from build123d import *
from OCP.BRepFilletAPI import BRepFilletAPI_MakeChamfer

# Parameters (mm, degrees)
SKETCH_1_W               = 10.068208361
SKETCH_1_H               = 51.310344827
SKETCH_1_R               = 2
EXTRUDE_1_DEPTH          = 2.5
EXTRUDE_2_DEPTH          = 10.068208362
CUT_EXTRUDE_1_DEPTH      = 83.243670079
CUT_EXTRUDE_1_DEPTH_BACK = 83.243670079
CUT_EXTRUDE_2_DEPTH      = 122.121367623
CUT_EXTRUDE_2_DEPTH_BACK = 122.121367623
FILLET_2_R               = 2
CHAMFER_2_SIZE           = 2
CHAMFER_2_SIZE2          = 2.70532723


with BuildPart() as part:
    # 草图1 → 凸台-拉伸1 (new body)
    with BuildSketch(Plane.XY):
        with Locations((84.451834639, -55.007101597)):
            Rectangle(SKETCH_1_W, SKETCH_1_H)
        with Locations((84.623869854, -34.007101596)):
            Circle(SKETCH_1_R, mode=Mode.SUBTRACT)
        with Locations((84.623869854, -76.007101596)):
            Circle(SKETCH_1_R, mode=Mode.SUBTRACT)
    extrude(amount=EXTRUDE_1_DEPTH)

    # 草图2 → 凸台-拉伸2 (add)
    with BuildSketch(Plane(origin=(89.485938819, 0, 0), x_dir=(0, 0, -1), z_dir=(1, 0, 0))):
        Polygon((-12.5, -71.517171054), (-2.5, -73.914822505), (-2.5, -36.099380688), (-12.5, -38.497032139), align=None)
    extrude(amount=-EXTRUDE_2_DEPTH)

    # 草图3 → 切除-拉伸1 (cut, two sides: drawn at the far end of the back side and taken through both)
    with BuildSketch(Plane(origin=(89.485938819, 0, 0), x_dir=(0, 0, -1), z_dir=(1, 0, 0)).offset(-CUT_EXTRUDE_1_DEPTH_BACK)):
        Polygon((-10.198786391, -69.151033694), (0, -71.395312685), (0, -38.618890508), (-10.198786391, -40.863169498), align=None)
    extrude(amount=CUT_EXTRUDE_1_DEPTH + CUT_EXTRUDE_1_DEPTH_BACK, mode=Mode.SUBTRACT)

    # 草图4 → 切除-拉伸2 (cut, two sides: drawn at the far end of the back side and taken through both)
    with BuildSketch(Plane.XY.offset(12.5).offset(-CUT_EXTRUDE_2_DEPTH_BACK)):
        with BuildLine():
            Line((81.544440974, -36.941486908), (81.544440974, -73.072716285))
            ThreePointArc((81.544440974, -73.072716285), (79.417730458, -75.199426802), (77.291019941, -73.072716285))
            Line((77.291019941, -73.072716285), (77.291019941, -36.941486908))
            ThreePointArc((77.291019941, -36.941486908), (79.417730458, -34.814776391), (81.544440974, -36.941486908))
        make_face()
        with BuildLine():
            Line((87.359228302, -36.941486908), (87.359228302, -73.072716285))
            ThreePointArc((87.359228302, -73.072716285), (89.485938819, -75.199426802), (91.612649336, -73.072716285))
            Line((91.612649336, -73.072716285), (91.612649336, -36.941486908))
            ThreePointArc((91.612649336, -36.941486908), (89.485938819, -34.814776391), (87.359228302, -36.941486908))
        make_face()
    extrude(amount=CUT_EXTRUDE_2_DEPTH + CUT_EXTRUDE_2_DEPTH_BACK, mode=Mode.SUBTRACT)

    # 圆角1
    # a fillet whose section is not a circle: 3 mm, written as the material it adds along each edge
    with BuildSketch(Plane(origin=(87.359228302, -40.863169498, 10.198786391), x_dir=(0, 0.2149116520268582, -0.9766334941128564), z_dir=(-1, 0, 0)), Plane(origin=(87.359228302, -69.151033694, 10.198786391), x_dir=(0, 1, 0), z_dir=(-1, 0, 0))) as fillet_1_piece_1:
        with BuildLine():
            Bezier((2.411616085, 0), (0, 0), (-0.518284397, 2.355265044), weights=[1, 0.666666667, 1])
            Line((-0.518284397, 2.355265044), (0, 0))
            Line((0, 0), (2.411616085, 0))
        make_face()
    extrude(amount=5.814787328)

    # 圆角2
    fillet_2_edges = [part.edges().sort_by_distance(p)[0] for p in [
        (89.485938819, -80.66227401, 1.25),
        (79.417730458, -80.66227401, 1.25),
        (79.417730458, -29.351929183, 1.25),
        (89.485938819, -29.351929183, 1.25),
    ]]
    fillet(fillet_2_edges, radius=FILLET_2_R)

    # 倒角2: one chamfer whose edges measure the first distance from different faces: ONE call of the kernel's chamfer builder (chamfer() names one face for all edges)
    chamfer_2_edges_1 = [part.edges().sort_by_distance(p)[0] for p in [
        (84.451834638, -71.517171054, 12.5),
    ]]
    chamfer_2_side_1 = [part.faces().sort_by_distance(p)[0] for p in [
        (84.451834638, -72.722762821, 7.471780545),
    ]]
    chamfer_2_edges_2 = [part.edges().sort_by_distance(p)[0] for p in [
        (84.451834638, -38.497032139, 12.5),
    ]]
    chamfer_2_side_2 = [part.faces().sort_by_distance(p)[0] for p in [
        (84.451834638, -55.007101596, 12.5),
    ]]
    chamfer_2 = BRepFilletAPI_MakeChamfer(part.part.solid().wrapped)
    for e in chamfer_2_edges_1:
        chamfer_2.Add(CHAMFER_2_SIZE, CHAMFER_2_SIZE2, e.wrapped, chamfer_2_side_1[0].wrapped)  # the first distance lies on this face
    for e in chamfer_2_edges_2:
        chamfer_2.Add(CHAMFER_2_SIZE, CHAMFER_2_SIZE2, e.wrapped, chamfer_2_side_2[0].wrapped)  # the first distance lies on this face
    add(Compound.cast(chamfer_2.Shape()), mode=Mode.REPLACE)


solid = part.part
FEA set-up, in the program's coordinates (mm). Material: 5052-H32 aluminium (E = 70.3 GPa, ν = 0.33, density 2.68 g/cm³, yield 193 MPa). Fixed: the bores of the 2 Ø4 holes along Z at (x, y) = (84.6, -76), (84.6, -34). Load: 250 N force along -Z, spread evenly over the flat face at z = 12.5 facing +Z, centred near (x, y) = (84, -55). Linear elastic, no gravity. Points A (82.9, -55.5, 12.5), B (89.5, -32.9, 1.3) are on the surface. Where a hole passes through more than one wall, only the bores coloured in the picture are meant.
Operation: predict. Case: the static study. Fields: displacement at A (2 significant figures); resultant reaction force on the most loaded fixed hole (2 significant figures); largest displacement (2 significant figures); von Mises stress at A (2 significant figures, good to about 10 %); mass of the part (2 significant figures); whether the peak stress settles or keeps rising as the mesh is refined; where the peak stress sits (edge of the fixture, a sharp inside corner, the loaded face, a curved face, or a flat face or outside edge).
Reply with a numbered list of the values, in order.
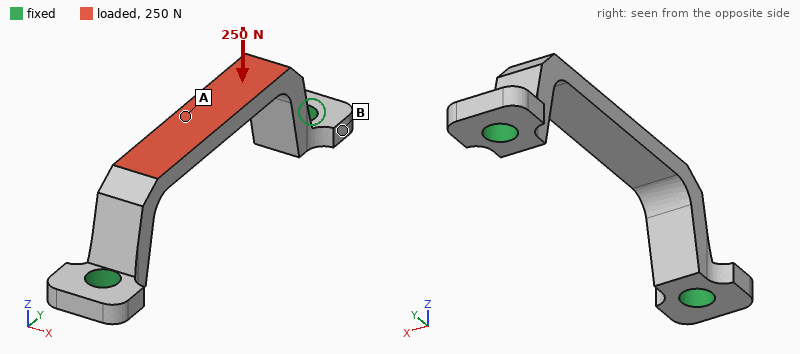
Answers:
1. 52 µm
2. 180 N
3. 53 µm
4. 74 MPa
5. 2.8 g
6. keeps rising
7. edge of the fixture
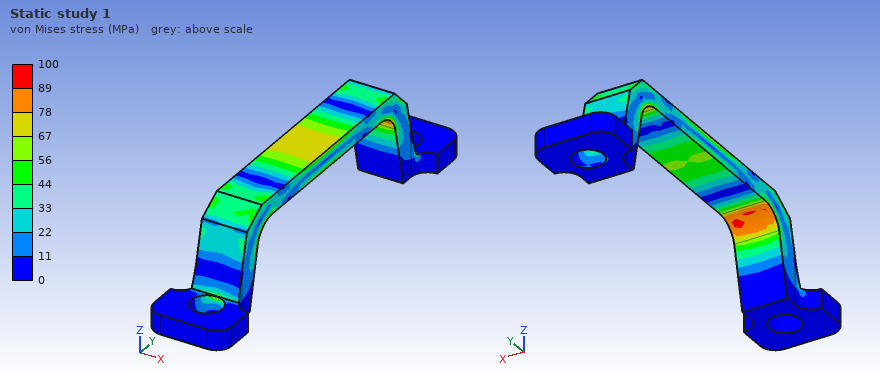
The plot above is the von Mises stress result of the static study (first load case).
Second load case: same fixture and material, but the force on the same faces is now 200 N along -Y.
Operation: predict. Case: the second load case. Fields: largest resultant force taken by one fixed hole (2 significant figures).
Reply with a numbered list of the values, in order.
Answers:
1. 100 N
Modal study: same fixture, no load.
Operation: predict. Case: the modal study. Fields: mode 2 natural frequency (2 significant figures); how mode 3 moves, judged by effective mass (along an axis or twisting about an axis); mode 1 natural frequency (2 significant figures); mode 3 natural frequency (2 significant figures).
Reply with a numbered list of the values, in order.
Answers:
1. 10 kHz
2. along Z
3. 10 kHz
4. 12 kHz
